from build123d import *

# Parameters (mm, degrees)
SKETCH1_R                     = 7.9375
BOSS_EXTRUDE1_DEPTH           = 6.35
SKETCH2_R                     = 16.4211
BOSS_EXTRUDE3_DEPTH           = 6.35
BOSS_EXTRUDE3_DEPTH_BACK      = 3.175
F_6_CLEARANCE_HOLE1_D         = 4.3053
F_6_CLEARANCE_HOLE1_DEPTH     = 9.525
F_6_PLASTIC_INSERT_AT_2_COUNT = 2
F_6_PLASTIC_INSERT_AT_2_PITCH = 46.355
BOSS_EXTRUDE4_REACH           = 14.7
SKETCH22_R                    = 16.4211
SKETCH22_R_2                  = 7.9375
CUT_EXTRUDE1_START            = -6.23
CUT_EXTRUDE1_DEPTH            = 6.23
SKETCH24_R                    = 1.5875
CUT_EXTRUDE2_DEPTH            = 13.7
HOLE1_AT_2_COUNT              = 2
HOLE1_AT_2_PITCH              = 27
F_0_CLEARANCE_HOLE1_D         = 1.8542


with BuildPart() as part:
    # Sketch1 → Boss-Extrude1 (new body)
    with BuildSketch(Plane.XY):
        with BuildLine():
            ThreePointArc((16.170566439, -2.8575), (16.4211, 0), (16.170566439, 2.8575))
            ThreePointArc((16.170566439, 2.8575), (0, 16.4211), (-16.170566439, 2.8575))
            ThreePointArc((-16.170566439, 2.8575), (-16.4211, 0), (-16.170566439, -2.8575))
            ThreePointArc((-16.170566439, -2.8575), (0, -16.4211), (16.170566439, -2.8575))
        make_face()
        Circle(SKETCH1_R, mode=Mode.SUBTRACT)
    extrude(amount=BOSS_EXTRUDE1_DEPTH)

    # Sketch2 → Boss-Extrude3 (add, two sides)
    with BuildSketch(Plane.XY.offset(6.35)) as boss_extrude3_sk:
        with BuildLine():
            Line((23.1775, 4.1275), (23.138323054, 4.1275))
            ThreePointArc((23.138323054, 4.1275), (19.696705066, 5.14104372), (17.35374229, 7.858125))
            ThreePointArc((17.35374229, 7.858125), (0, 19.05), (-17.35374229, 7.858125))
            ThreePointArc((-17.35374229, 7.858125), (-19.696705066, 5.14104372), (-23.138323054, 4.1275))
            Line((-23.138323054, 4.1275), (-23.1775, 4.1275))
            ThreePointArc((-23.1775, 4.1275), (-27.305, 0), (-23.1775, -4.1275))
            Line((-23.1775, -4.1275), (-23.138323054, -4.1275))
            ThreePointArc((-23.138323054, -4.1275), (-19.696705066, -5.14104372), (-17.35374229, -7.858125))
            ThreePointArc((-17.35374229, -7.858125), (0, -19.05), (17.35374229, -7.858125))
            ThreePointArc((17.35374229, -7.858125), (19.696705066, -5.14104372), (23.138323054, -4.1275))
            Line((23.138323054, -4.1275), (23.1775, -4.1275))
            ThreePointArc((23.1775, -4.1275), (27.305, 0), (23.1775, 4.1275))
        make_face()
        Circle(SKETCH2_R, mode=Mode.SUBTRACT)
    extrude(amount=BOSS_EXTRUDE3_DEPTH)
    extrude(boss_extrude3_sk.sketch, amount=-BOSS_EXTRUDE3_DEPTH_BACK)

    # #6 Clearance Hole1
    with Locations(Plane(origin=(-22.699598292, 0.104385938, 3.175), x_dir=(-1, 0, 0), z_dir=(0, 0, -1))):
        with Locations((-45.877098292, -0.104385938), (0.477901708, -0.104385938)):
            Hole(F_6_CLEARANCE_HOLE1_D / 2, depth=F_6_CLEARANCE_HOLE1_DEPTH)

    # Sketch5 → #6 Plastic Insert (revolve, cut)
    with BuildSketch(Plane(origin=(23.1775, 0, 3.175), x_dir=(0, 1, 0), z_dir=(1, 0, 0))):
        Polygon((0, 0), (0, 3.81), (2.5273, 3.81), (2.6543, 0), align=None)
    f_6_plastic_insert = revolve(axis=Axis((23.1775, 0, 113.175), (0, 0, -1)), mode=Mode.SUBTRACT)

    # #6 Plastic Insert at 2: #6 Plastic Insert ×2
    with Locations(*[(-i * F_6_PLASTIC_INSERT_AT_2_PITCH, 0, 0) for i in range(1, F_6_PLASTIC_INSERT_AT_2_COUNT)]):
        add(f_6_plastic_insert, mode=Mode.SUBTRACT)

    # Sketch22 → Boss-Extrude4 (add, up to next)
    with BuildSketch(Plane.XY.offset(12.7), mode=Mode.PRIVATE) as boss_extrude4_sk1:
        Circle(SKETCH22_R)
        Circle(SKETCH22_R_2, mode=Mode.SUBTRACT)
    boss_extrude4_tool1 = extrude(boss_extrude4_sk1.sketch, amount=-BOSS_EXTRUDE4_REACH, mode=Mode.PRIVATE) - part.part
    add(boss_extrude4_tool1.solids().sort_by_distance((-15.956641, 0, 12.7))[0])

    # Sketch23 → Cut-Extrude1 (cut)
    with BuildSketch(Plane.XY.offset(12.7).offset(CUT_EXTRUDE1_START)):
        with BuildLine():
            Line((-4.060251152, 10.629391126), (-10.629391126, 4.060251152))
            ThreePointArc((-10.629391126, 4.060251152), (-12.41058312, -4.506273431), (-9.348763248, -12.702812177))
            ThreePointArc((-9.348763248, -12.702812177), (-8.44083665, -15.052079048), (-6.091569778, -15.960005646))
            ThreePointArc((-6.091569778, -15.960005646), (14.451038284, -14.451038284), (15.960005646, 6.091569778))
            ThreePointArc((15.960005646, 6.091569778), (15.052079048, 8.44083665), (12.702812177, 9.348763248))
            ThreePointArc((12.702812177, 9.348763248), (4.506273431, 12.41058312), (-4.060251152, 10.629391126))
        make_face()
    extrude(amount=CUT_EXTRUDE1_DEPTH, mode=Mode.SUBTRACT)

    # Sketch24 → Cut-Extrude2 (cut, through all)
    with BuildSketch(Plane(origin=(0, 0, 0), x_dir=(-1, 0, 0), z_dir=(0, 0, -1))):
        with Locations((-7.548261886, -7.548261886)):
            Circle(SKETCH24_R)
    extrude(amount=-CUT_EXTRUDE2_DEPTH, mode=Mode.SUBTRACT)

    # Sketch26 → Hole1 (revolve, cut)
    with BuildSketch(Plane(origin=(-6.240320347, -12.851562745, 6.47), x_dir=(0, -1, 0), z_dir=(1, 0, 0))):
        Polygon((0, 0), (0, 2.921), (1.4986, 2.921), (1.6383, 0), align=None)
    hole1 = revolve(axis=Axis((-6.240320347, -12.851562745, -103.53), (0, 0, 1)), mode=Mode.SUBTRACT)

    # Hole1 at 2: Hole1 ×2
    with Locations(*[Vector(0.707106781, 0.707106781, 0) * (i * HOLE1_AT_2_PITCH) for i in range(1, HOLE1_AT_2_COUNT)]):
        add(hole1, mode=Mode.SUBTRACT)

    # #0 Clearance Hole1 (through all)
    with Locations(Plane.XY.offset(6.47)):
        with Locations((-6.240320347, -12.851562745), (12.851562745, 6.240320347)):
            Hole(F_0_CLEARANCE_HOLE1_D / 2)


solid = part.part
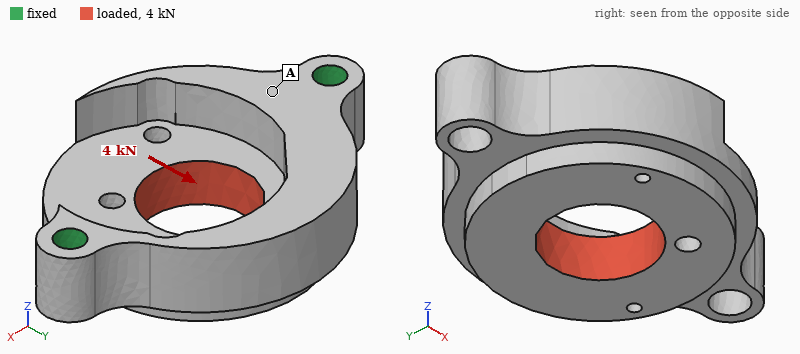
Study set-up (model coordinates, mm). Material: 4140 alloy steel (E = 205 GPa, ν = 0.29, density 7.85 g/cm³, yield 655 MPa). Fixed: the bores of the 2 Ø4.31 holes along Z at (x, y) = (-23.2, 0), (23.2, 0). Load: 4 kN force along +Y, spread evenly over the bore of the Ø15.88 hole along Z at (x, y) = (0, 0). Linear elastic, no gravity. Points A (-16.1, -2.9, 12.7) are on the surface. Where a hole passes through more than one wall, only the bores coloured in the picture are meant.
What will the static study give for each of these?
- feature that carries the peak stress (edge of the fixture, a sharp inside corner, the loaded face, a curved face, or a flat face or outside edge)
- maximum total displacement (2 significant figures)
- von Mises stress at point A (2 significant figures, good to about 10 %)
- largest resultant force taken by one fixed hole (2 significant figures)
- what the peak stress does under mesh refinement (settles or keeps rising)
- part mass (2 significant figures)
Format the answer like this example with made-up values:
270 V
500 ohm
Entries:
edge of the fixture
33 µm
37 MPa
2.0 kN
keeps rising
66 g
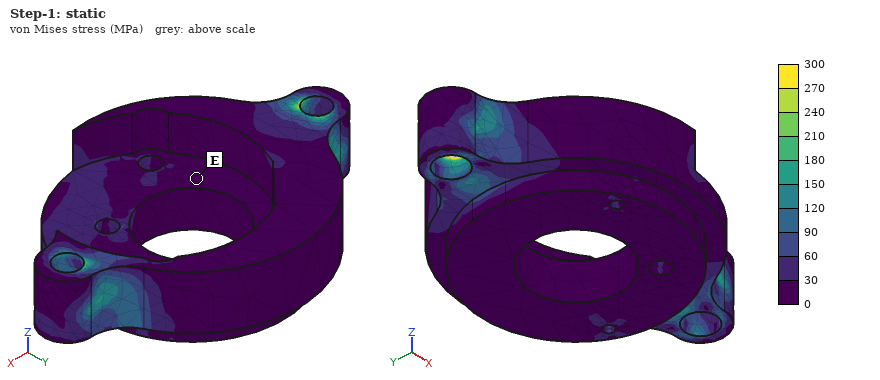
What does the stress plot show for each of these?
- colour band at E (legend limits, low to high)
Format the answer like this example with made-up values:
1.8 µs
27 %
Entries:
0 to 30 MPa
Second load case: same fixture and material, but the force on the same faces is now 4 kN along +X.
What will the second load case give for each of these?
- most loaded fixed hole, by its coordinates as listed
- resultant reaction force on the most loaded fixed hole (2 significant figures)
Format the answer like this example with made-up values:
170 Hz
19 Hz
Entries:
(-23.2, 0)
2.3 kN
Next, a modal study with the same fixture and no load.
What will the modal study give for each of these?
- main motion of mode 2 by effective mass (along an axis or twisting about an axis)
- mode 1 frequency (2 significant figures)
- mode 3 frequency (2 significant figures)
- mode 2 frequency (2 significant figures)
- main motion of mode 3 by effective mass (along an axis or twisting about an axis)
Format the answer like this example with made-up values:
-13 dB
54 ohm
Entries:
along Z
6900 Hz
18 kHz
11 kHz
along Y
